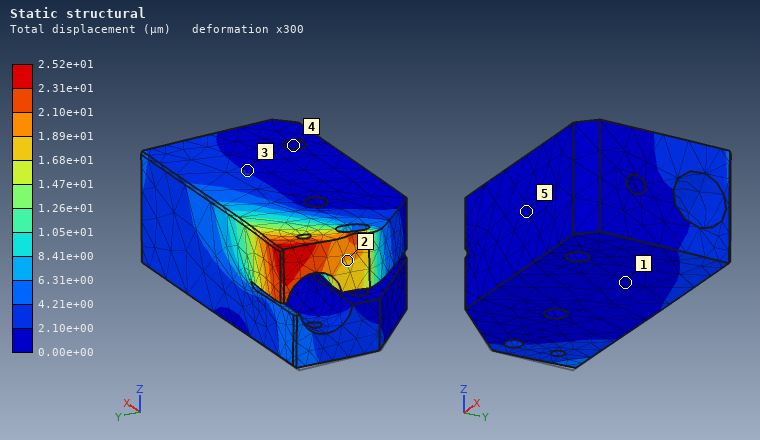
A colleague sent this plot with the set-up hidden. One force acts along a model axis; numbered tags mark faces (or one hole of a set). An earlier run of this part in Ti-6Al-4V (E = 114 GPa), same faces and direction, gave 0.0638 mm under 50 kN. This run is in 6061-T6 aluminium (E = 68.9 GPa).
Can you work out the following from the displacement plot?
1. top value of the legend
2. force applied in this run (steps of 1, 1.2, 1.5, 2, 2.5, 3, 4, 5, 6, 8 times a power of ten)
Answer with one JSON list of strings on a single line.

["2.52e+01 µm", "12 kN"]
